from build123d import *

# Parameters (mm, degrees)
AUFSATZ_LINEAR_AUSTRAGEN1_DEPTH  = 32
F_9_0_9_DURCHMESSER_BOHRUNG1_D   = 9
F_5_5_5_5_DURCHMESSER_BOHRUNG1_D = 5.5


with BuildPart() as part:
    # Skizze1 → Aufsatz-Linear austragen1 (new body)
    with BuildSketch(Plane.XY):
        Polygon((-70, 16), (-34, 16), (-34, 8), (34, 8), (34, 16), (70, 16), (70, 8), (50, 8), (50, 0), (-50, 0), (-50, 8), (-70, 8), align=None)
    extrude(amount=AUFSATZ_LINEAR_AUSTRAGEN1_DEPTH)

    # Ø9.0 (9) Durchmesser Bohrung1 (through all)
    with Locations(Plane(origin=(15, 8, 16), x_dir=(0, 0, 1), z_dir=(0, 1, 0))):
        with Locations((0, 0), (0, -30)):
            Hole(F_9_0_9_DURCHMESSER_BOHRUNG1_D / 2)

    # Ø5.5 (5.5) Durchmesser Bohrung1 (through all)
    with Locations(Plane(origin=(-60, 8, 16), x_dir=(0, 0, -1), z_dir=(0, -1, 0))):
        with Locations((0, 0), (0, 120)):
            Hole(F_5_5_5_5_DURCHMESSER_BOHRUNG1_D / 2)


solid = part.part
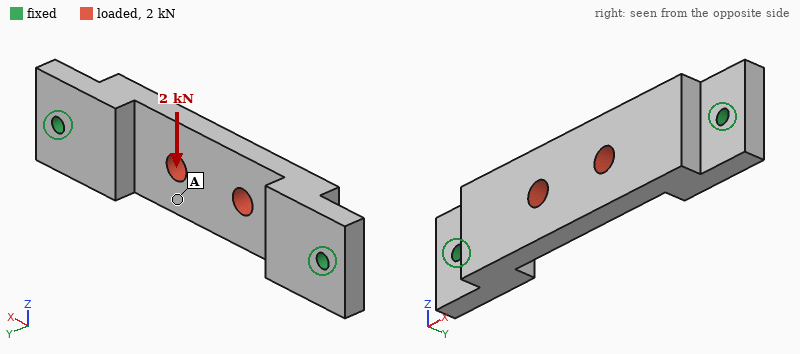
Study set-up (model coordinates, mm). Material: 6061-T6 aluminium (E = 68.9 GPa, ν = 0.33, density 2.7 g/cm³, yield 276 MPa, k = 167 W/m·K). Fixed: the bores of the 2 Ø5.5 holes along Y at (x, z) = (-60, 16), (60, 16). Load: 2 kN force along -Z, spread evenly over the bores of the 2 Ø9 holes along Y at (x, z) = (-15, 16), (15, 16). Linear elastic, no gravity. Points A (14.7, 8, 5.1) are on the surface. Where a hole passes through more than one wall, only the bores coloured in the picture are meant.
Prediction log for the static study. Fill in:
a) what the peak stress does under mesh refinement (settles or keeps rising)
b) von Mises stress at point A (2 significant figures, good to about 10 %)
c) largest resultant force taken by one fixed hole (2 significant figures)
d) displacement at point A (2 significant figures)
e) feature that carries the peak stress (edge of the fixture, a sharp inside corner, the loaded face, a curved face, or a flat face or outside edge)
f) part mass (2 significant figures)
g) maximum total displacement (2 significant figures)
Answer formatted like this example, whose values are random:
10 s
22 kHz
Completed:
keeps rising
16 MPa
1.0 kN
37 µm
edge of the fixture
120 g
49 µm
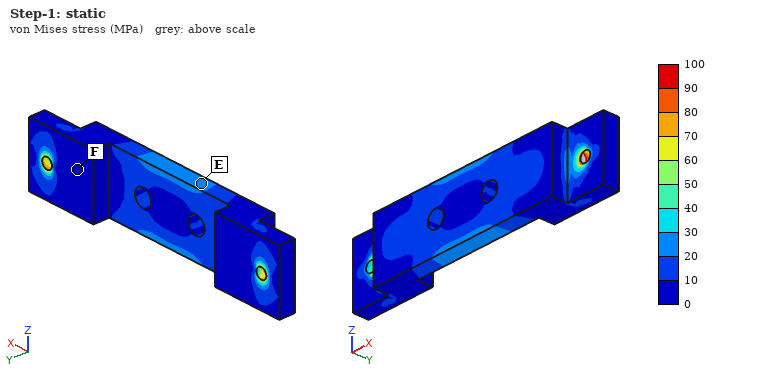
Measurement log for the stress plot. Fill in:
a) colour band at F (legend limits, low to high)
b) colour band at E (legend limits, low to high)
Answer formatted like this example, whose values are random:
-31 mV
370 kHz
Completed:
0 to 10 MPa
20 to 30 MPa
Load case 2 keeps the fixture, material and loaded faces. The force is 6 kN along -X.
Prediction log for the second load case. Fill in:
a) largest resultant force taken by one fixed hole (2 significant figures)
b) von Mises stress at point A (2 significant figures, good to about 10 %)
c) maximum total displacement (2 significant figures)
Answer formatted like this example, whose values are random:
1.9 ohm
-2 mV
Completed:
3.0 kN
23 MPa
29 µm
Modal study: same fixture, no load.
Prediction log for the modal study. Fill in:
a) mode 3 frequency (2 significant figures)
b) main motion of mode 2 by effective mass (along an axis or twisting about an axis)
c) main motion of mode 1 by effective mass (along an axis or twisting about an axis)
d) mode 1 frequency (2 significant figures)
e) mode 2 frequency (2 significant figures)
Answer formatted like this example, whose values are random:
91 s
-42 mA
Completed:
6100 Hz
along Z
along Y
4000 Hz
4600 Hz
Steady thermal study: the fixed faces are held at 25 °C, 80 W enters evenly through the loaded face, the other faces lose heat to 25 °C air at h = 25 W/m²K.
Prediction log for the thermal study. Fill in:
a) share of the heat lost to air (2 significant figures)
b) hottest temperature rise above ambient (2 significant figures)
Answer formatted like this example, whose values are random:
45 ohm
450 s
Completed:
8.2 %
44 K
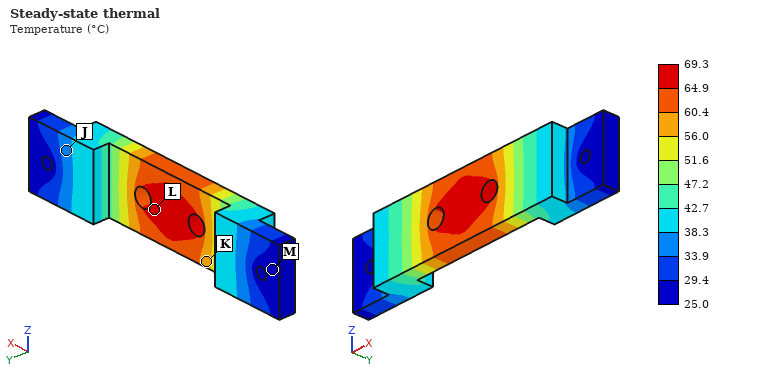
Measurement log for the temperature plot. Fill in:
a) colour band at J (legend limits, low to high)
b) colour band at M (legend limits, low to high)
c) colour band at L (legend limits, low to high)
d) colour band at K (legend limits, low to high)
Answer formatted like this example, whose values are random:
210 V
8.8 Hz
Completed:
33.9 to 38.3 °C
25.0 to 29.4 °C
64.9 to 69.3 °C
56.0 to 60.4 °C
